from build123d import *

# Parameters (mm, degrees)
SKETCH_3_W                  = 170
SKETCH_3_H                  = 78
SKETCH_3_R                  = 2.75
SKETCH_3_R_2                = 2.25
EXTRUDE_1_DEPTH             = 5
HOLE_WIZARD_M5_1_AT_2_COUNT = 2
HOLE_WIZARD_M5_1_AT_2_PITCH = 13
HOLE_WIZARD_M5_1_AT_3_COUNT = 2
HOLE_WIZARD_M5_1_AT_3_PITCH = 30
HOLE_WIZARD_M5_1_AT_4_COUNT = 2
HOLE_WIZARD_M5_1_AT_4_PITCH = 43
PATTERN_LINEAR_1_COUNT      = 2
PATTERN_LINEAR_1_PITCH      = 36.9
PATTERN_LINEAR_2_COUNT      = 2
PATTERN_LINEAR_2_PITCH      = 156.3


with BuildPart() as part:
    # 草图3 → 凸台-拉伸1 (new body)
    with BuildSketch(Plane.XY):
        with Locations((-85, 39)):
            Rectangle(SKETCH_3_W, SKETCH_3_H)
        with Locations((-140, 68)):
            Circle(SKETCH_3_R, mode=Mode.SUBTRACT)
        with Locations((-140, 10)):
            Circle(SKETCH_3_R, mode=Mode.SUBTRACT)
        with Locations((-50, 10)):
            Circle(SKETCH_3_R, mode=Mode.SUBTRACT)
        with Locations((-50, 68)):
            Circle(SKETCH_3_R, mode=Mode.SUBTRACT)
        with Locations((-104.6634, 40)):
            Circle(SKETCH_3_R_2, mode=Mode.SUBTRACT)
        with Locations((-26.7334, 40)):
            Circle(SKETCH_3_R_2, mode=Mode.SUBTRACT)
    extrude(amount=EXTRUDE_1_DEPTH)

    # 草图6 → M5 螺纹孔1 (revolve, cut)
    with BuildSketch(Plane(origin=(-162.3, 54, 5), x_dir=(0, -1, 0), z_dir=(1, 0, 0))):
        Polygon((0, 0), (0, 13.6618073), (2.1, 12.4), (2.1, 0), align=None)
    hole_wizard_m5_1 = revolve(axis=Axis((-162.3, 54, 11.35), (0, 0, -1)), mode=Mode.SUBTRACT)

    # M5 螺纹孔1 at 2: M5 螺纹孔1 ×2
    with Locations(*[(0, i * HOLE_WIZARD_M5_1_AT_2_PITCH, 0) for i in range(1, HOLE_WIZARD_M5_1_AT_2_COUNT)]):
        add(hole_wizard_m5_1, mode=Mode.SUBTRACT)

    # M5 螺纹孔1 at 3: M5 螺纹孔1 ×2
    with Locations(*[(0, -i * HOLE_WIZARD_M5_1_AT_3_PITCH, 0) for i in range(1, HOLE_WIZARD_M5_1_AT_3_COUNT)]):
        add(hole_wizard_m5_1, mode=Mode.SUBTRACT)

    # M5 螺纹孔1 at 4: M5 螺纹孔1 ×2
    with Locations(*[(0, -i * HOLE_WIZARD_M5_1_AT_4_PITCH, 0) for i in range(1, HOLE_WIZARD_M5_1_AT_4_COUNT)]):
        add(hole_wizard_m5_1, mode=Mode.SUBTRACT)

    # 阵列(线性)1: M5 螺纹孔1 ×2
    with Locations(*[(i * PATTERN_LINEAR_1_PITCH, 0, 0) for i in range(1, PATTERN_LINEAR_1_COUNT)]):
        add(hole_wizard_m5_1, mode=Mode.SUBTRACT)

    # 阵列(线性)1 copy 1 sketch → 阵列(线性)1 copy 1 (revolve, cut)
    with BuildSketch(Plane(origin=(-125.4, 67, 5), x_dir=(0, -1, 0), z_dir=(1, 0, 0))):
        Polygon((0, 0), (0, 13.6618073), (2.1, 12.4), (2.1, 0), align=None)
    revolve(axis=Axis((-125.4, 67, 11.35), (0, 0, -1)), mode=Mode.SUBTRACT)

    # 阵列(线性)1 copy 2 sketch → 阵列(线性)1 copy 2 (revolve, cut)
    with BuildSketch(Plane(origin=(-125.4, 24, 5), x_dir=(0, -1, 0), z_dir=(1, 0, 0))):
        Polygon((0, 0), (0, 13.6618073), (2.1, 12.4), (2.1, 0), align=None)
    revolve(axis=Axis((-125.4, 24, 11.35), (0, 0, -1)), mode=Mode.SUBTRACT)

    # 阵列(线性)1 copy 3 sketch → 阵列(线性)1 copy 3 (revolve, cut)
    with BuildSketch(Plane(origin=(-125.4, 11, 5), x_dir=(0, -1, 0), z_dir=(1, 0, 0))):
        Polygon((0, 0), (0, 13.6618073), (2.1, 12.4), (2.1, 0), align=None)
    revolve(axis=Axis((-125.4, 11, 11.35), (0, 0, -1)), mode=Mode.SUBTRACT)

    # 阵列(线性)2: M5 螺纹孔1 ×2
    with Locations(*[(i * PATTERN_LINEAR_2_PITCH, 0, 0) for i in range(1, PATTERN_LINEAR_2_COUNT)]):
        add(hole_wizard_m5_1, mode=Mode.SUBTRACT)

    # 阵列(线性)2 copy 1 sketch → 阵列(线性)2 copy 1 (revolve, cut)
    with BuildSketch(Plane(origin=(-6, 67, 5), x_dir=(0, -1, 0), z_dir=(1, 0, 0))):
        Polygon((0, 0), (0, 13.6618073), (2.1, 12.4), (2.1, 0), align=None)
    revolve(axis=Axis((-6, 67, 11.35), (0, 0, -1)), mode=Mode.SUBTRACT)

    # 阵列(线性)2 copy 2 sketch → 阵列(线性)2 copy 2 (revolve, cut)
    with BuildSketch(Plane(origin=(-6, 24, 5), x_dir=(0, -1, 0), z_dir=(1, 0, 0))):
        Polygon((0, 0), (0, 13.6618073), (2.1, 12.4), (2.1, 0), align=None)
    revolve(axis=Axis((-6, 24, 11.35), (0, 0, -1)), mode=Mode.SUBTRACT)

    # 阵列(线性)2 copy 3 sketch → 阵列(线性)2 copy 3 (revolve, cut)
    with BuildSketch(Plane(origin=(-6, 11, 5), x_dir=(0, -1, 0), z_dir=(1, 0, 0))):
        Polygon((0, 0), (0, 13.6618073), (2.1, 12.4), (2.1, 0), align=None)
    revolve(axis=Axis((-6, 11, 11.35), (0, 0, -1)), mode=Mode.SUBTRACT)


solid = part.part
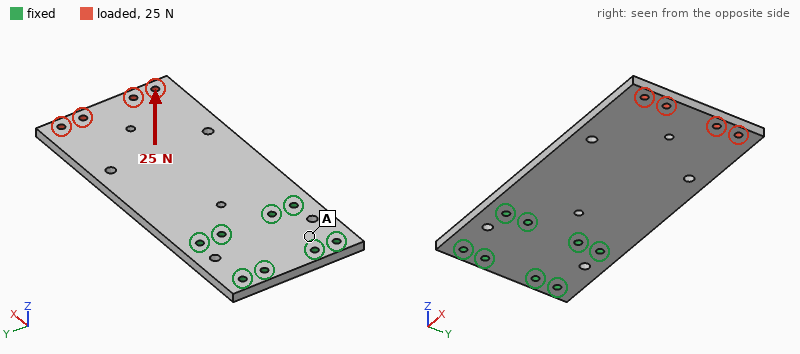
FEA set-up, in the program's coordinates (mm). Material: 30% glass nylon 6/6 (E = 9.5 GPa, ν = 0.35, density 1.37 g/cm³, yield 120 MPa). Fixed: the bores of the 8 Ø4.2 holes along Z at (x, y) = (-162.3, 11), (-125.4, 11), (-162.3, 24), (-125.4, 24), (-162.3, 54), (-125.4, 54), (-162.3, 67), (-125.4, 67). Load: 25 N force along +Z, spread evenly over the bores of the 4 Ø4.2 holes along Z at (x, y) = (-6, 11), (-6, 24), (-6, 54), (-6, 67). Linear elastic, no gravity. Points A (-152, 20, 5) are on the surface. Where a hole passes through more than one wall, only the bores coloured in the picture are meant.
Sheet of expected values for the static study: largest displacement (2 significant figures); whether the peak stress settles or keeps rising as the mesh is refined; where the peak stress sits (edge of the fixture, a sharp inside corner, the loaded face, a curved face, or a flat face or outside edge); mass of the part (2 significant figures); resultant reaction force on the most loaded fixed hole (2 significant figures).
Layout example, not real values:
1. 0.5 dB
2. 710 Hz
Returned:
1. 1.9 mm
2. keeps rising
3. edge of the fixture
4. 89 g
5. 28 N
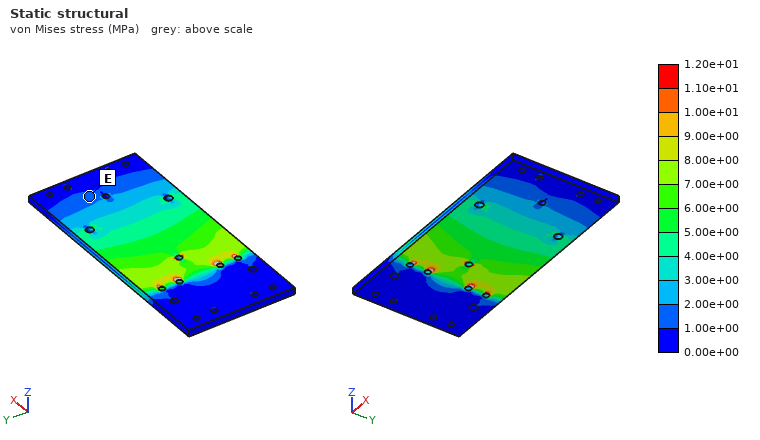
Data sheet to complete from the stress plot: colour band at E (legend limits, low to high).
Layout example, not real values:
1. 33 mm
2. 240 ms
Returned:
1. 1.00e+00 to 2.00e+00 MPa
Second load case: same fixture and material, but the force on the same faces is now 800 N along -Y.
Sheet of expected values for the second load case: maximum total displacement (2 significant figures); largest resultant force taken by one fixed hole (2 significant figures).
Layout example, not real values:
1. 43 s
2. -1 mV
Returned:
1. 0.40 mm
2. 1.2 kN
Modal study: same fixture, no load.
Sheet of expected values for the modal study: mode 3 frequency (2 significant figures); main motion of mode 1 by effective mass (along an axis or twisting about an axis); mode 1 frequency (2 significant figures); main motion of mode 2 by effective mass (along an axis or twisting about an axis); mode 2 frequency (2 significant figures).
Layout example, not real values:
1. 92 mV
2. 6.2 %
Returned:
1. 860 Hz
2. along Z
3. 140 Hz
4. twisting about X
5. 480 Hz
